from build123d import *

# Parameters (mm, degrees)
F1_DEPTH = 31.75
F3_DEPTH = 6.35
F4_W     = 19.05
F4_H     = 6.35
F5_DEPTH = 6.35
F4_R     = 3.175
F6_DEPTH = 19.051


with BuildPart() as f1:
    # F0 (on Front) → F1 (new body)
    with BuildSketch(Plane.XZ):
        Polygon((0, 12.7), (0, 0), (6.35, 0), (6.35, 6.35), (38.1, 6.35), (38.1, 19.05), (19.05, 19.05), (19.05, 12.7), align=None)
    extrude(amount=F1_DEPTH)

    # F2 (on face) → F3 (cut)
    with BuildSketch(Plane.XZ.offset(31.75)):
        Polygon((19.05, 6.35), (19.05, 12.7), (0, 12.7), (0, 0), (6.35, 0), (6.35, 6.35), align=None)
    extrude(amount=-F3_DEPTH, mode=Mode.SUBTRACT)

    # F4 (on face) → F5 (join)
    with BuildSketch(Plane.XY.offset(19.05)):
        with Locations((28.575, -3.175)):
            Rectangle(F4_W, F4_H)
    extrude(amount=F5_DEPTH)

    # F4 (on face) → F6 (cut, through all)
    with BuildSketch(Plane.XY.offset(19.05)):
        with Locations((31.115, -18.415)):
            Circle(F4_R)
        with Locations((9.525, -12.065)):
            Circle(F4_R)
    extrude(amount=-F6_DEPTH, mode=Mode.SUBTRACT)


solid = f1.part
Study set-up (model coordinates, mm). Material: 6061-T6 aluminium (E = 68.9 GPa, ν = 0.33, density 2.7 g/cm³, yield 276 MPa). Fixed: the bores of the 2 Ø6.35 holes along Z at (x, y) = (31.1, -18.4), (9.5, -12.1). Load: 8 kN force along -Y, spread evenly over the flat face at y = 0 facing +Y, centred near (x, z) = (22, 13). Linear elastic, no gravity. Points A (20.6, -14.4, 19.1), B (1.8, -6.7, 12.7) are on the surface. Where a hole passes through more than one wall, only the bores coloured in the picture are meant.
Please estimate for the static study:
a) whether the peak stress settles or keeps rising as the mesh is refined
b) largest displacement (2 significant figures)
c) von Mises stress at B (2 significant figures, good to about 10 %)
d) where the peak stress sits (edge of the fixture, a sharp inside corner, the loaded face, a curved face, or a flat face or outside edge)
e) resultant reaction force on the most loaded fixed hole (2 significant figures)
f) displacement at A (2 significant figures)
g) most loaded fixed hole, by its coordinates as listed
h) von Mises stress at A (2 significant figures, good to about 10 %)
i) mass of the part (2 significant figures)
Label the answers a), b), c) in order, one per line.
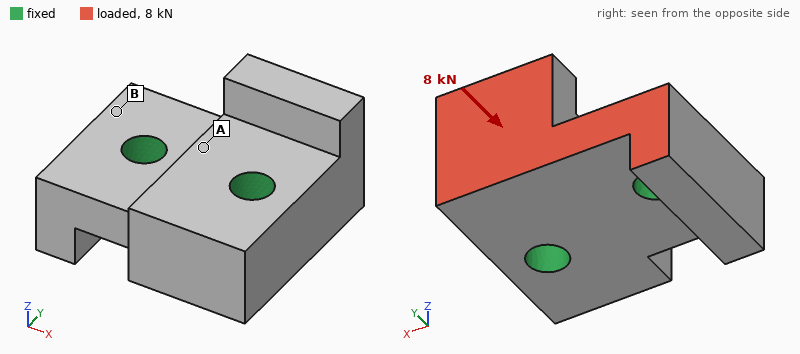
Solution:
a) keeps rising
b) 32 µm
c) 12 MPa
d) edge of the fixture
e) 5.1 kN
f) 6.0 µm
g) (31.1, -18.4)
h) 28 MPa
i) 32 g
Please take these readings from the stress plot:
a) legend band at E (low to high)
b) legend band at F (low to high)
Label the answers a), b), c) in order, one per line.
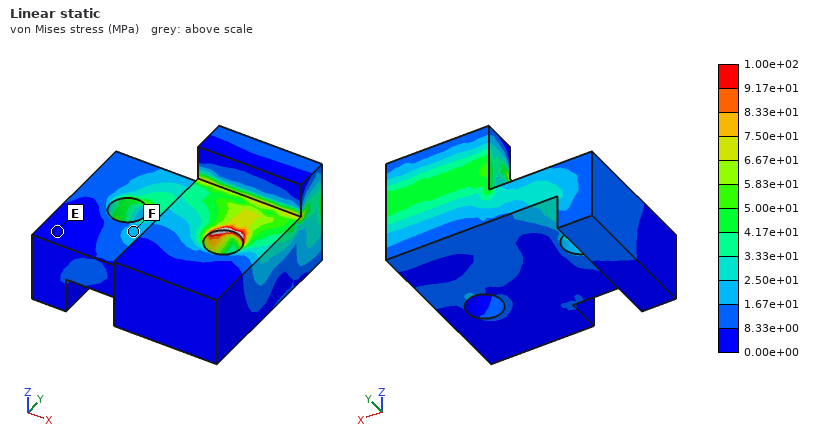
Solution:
a) 0.00e+00 to 8.33e+00 MPa
b) 1.67e+01 to 2.50e+01 MPa
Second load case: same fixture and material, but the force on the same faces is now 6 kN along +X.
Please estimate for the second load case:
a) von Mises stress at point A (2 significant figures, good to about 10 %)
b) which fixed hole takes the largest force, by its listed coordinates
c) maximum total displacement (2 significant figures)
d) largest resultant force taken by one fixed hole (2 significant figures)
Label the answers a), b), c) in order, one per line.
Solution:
a) 26 MPa
b) (9.5, -12.1)
c) 36 µm
d) 4.6 kN
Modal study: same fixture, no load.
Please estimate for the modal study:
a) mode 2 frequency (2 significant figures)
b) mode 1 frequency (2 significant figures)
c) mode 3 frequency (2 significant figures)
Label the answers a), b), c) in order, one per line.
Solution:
a) 24 kHz
b) 21 kHz
c) 27 kHz
